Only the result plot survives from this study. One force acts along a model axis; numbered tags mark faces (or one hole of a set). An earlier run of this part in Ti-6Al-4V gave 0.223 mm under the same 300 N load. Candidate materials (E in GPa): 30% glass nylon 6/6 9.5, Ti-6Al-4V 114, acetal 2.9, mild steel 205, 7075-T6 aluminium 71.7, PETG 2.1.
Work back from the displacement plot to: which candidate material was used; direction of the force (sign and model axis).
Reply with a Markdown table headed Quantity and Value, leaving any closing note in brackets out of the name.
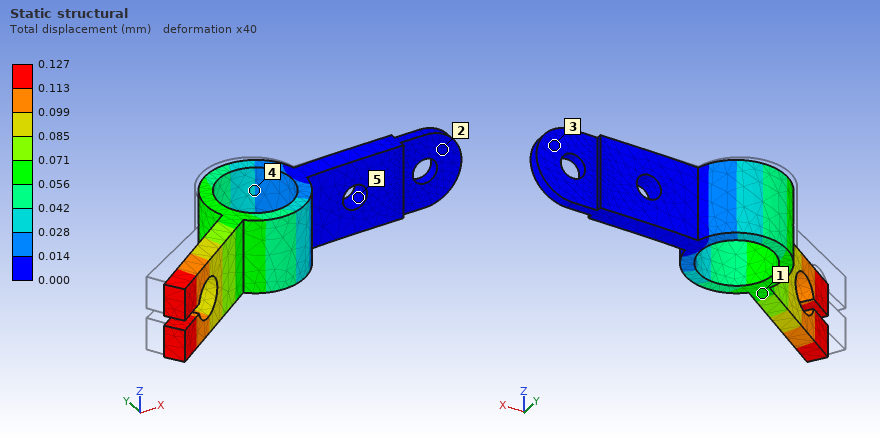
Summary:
| Quantity | Value |
|---|---|
| which candidate material was used | mild steel |
| direction of the force | -Y |
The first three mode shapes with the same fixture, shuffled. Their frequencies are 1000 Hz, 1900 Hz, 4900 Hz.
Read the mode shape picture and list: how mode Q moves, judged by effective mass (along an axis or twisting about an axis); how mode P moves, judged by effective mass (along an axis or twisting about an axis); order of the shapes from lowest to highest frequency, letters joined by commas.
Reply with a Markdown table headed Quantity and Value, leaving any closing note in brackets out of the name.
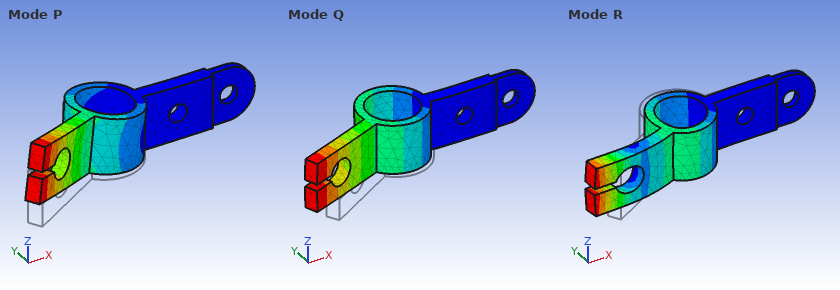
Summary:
| Quantity | Value |
|---|---|
| how mode Q moves, judged by effective mass | along Y |
| how mode P moves, judged by effective mass | along Z |
| order of the shapes from lowest to highest frequency, letters joined by commas | Q, P, R |
